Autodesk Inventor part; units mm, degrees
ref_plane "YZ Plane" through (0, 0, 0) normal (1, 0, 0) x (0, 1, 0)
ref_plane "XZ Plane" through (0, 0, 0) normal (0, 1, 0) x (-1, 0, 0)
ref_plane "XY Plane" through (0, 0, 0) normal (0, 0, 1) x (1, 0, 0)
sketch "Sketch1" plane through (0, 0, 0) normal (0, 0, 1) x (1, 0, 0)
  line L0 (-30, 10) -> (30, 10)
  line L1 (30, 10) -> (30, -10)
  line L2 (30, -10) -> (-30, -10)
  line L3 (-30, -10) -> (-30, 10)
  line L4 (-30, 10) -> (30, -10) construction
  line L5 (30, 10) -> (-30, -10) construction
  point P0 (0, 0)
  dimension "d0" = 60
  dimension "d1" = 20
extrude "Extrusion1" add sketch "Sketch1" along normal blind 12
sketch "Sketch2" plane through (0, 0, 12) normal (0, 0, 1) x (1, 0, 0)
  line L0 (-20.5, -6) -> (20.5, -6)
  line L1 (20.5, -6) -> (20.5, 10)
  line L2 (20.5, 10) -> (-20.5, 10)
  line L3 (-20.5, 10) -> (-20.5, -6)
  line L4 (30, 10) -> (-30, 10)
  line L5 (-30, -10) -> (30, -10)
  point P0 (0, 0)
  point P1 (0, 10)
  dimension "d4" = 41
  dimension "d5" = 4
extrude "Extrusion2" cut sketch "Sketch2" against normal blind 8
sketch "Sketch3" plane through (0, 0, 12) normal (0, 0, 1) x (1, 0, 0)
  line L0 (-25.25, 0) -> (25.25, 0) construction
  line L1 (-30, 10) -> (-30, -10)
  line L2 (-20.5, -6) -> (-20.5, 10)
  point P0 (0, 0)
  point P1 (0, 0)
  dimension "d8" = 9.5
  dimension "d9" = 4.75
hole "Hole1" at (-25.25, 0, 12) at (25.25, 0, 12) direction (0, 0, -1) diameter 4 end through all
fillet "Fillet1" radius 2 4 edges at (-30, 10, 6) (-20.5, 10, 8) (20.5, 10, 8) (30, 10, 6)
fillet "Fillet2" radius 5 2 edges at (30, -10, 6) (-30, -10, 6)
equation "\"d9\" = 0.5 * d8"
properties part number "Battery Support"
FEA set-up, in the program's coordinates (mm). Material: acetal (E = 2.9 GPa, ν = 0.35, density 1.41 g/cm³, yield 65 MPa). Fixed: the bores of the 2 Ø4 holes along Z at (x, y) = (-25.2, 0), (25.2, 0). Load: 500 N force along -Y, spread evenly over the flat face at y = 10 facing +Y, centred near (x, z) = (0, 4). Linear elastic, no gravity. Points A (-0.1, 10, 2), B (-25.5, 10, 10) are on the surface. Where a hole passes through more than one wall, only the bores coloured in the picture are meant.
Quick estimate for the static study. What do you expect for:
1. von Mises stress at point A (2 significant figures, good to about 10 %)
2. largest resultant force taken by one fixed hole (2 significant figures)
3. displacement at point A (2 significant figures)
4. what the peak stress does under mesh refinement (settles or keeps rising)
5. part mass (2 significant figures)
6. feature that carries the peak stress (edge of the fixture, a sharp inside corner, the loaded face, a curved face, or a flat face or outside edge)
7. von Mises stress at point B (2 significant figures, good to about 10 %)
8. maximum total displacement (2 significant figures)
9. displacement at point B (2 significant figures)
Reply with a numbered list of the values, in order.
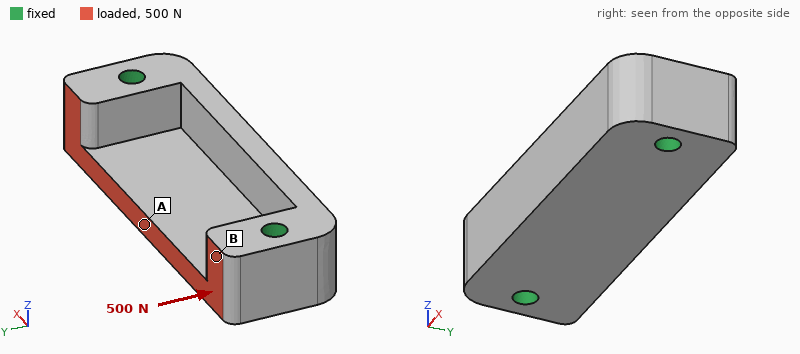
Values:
1. 3.8 MPa
2. 250 N
3. 52 µm
4. keeps rising
5. 12 g
6. edge of the fixture
7. 1.4 MPa
8. 53 µm
9. 11 µm
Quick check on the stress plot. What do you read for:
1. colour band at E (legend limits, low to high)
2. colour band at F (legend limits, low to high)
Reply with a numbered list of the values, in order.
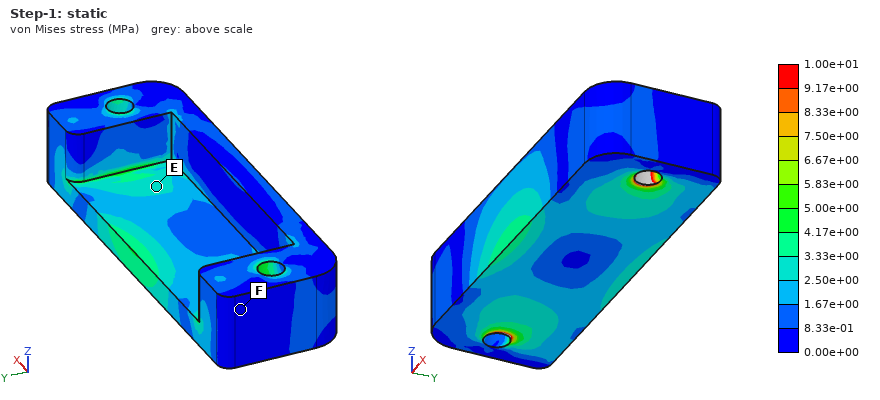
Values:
1. 2.50e+00 to 3.33e+00 MPa
2. 0.00e+00 to 8.33e-01 MPa
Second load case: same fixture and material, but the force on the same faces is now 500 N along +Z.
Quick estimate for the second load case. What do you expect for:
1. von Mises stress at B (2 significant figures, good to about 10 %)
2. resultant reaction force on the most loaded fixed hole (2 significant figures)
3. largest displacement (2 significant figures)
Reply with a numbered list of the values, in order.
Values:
1. 4.0 MPa
2. 250 N
3. 0.51 mm
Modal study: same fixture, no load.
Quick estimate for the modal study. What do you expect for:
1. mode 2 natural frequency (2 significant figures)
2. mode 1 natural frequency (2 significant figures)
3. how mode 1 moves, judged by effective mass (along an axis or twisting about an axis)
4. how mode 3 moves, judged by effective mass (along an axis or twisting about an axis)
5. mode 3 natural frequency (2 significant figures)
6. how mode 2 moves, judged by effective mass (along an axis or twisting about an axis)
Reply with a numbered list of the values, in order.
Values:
1. 4400 Hz
2. 3400 Hz
3. along Z
4. along Y
5. 5600 Hz
6. along Y
